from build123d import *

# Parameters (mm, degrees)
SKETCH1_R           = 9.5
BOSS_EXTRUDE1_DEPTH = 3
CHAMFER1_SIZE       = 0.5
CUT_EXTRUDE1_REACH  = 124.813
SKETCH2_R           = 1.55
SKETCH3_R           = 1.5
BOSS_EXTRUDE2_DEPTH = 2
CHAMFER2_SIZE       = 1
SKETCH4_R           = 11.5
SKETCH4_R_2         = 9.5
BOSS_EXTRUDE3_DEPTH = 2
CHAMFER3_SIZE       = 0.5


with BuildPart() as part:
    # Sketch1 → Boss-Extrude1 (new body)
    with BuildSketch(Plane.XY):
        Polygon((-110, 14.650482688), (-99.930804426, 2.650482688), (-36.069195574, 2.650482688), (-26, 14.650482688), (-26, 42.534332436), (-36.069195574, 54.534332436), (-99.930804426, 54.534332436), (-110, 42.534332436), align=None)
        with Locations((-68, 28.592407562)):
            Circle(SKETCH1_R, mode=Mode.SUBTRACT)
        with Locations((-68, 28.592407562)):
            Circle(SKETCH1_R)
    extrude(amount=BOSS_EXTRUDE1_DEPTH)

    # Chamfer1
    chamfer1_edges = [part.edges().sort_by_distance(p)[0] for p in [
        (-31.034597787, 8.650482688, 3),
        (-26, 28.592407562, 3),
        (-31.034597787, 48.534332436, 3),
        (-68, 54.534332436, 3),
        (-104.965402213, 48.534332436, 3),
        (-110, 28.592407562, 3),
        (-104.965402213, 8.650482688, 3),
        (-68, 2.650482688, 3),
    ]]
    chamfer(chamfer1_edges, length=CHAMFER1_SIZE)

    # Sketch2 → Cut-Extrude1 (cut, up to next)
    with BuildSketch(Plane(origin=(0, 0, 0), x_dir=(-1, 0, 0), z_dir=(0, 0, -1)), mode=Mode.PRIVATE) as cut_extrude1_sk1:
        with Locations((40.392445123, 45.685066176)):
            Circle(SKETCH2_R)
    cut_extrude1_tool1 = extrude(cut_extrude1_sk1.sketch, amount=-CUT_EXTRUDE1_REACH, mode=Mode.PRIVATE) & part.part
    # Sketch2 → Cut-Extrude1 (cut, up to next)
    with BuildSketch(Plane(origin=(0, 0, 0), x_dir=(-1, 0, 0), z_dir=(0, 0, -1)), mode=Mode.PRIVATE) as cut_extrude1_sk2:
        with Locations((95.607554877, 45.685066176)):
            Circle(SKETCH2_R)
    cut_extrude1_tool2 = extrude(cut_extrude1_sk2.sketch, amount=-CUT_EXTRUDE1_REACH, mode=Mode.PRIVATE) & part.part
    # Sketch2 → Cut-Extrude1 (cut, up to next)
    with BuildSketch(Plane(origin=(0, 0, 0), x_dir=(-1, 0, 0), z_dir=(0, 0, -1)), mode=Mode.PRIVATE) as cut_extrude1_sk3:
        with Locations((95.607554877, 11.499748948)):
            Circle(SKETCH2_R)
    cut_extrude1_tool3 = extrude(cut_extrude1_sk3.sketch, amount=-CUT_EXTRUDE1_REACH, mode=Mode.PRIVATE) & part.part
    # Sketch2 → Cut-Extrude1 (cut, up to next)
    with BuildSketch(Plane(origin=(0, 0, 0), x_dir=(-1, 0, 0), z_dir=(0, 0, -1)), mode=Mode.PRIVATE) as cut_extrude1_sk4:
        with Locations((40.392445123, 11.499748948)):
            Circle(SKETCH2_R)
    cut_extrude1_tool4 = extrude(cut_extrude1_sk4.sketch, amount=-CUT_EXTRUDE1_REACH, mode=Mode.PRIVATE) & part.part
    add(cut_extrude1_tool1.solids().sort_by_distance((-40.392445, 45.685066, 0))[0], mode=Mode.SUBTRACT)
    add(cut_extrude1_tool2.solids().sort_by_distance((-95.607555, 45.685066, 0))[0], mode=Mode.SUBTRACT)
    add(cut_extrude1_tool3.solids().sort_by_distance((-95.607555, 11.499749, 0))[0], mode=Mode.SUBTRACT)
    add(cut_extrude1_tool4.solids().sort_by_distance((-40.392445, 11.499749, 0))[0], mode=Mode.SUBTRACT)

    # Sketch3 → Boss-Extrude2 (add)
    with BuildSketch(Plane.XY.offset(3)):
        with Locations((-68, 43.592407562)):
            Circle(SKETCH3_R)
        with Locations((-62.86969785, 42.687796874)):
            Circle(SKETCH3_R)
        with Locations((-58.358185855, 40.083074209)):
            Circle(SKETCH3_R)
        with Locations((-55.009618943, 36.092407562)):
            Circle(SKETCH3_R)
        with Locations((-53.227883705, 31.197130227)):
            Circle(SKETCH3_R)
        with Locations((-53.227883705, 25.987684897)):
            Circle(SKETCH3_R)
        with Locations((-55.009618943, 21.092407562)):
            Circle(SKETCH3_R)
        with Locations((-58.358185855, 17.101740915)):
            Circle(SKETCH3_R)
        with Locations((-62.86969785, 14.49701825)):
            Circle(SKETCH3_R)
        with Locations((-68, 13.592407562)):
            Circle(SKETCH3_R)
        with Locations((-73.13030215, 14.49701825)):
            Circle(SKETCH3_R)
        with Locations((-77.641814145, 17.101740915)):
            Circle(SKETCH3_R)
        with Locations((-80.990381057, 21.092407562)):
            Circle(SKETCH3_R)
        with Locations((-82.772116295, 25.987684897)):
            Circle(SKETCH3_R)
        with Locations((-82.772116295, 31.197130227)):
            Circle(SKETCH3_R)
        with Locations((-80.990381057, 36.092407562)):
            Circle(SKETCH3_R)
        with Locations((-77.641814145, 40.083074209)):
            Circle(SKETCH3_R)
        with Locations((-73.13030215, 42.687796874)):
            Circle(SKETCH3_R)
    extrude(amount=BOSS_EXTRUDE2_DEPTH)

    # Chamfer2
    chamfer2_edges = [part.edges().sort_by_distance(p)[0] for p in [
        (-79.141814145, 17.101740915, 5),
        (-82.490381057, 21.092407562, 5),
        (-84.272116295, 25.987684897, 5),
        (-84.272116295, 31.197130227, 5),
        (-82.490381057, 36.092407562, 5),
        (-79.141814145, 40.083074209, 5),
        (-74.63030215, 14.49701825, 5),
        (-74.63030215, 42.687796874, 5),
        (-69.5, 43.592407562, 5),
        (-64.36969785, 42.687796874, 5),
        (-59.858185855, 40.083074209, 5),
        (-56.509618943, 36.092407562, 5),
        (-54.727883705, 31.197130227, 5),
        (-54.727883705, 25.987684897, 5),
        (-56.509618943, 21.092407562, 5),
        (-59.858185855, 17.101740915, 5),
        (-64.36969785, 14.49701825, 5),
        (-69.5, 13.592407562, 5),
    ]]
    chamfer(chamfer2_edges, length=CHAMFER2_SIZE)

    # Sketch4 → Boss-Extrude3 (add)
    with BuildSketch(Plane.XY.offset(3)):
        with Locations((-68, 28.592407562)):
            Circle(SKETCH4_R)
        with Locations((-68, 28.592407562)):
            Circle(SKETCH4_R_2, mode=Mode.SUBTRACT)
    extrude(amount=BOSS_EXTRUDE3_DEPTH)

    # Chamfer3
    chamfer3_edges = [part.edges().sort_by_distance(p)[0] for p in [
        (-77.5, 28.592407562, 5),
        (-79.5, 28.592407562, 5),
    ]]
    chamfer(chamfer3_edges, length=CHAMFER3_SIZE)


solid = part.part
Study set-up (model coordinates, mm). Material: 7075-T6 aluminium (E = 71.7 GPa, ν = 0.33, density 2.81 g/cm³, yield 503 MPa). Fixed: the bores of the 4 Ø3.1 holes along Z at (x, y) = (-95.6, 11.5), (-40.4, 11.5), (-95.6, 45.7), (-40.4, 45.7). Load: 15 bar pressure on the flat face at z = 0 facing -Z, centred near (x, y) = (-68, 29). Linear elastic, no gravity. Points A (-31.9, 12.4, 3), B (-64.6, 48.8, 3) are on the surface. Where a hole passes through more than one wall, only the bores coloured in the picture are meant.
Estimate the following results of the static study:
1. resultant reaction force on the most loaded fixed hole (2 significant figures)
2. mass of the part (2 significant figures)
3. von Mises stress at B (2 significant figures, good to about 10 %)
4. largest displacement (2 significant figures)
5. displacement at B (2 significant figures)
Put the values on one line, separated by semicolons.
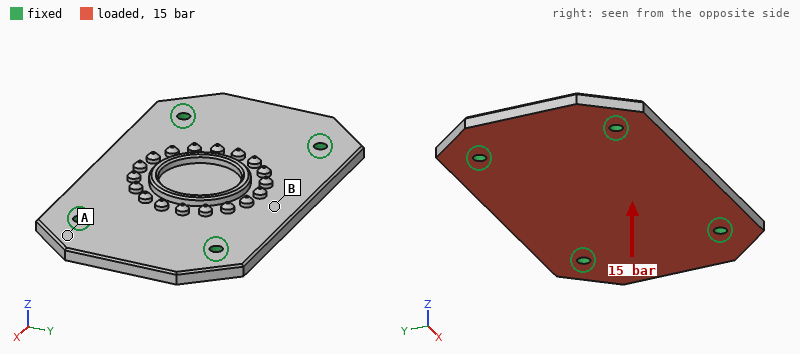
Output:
1.5 kN; 36 g; 120 MPa; 0.26 mm; 0.24 mm
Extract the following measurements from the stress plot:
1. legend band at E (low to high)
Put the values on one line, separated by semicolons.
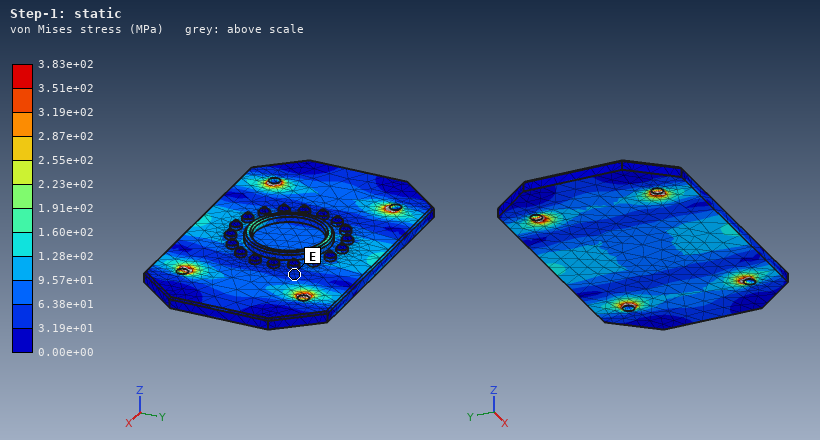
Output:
3.19e+01 to 6.38e+01 MPa
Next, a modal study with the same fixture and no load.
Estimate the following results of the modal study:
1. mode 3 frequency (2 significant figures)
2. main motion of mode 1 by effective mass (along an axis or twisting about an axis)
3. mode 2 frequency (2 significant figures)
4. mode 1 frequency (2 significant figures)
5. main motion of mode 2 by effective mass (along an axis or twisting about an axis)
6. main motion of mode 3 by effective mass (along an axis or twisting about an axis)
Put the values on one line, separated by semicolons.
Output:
8700 Hz; along Z; 5900 Hz; 4500 Hz; twisting about X; along Z
